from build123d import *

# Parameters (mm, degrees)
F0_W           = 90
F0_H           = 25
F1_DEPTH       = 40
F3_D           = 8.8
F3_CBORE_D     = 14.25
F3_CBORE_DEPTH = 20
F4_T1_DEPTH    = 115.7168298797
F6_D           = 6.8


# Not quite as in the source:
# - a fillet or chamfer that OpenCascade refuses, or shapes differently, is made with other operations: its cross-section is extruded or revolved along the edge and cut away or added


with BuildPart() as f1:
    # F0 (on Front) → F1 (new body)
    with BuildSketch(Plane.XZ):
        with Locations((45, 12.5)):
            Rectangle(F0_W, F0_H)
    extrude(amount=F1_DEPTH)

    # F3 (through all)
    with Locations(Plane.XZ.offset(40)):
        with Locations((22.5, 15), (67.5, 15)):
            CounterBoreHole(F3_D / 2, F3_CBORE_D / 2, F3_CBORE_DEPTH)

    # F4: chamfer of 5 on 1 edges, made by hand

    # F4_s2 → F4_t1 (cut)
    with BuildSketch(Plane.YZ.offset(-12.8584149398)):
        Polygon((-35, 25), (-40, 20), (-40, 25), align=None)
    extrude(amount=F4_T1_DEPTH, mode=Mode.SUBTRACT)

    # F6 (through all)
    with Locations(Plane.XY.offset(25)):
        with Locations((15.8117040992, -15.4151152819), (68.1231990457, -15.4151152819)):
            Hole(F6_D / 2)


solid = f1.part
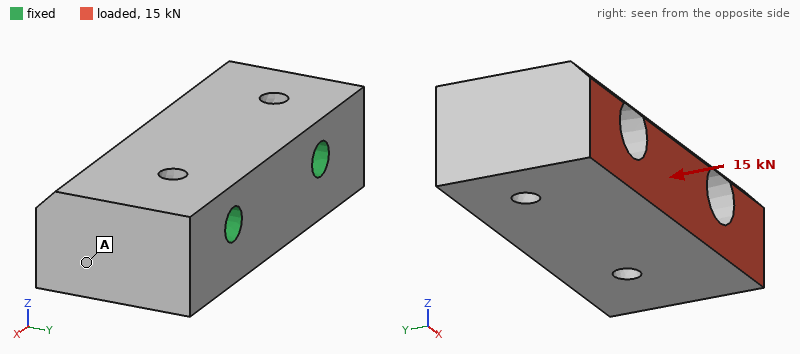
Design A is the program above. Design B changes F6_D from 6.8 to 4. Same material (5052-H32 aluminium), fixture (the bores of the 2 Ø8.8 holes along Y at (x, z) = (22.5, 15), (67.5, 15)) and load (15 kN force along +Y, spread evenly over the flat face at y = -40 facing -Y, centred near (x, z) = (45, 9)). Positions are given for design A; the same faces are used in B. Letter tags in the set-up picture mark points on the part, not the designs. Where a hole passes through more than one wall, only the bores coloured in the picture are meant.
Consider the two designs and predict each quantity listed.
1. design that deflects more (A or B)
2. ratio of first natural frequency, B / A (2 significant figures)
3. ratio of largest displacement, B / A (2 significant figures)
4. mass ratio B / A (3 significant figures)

A
1.1
0.90
1.01
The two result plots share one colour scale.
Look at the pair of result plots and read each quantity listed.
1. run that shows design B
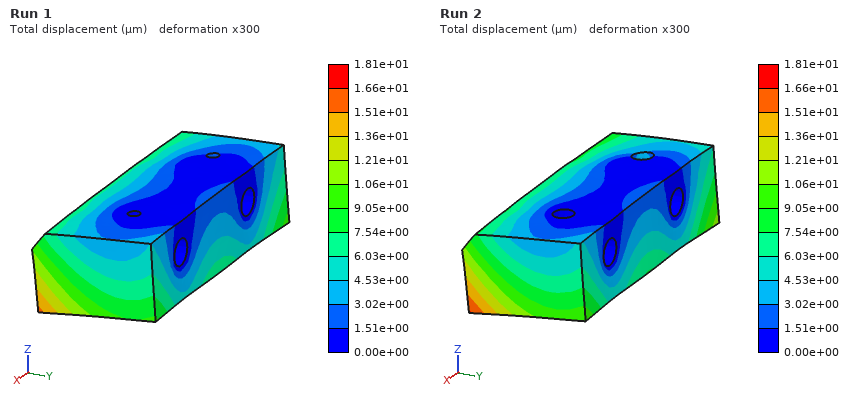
Run 1
